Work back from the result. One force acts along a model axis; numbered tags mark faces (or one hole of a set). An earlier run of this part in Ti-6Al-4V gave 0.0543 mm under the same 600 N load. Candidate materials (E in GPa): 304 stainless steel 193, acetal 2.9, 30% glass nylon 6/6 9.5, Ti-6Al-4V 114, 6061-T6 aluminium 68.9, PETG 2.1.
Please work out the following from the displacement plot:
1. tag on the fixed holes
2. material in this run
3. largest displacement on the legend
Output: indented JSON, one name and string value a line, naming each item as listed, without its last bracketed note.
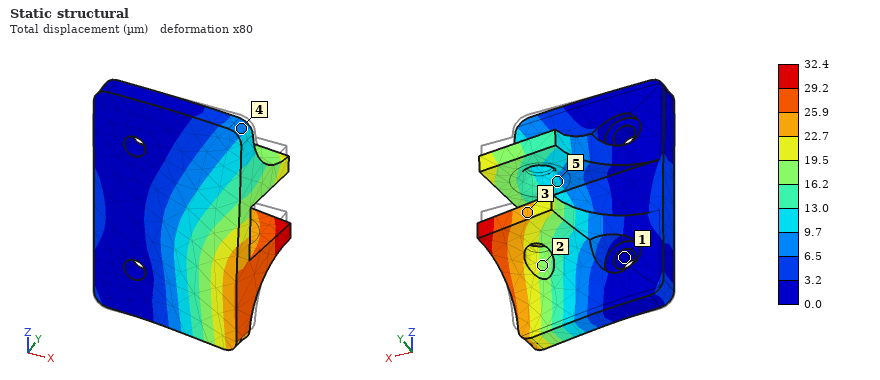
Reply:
{
  "tag on the fixed holes": "1",
  "material in this run": "304 stainless steel",
  "largest displacement on the legend": "32.4 µm"
}
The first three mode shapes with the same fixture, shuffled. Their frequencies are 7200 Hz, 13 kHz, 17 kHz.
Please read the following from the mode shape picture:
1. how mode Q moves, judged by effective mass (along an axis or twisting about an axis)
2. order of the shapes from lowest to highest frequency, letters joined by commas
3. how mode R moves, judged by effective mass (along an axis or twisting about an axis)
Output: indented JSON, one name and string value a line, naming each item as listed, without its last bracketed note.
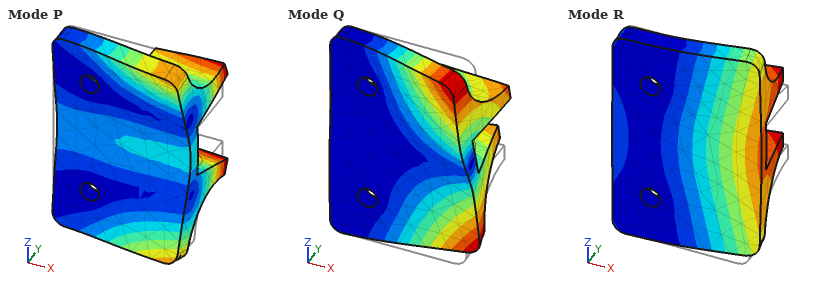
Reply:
{
  "how mode Q moves, judged by effective mass": "twisting about X",
  "order of the shapes from lowest to highest frequency, letters joined by commas": "R, Q, P",
  "how mode R moves, judged by effective mass": "along Y"
}
